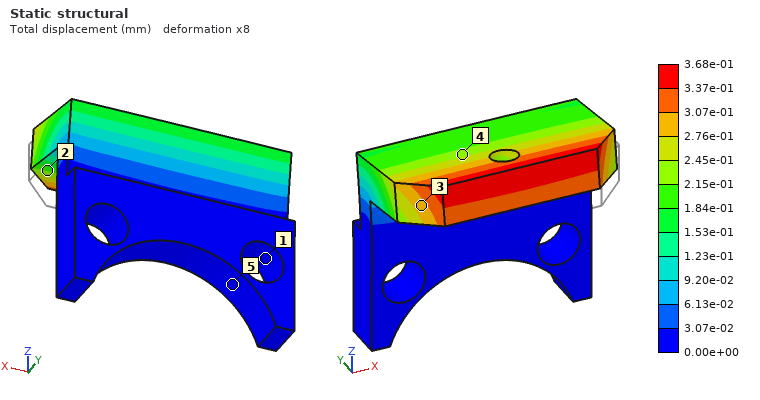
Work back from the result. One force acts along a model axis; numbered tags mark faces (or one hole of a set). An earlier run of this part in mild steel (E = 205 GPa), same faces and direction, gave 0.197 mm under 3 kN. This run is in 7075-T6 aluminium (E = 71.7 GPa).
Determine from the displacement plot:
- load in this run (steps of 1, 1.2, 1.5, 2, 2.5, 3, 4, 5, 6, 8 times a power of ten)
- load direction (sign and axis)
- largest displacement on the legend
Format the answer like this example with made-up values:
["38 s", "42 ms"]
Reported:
["2 kN", "+Z", "3.68e-01 mm"]
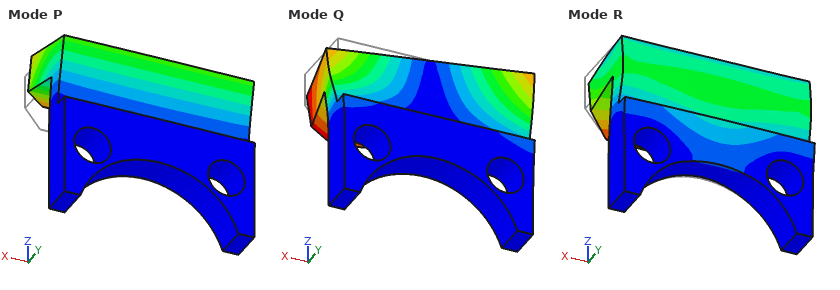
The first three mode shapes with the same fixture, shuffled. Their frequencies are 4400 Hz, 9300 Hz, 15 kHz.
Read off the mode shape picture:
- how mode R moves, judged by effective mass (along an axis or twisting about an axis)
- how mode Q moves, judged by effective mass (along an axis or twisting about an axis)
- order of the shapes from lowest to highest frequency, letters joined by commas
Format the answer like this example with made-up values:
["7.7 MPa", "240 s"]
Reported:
["along Y", "along X", "P, Q, R"]
